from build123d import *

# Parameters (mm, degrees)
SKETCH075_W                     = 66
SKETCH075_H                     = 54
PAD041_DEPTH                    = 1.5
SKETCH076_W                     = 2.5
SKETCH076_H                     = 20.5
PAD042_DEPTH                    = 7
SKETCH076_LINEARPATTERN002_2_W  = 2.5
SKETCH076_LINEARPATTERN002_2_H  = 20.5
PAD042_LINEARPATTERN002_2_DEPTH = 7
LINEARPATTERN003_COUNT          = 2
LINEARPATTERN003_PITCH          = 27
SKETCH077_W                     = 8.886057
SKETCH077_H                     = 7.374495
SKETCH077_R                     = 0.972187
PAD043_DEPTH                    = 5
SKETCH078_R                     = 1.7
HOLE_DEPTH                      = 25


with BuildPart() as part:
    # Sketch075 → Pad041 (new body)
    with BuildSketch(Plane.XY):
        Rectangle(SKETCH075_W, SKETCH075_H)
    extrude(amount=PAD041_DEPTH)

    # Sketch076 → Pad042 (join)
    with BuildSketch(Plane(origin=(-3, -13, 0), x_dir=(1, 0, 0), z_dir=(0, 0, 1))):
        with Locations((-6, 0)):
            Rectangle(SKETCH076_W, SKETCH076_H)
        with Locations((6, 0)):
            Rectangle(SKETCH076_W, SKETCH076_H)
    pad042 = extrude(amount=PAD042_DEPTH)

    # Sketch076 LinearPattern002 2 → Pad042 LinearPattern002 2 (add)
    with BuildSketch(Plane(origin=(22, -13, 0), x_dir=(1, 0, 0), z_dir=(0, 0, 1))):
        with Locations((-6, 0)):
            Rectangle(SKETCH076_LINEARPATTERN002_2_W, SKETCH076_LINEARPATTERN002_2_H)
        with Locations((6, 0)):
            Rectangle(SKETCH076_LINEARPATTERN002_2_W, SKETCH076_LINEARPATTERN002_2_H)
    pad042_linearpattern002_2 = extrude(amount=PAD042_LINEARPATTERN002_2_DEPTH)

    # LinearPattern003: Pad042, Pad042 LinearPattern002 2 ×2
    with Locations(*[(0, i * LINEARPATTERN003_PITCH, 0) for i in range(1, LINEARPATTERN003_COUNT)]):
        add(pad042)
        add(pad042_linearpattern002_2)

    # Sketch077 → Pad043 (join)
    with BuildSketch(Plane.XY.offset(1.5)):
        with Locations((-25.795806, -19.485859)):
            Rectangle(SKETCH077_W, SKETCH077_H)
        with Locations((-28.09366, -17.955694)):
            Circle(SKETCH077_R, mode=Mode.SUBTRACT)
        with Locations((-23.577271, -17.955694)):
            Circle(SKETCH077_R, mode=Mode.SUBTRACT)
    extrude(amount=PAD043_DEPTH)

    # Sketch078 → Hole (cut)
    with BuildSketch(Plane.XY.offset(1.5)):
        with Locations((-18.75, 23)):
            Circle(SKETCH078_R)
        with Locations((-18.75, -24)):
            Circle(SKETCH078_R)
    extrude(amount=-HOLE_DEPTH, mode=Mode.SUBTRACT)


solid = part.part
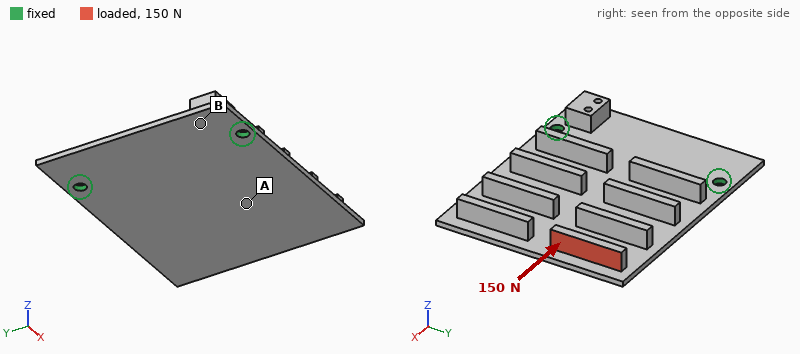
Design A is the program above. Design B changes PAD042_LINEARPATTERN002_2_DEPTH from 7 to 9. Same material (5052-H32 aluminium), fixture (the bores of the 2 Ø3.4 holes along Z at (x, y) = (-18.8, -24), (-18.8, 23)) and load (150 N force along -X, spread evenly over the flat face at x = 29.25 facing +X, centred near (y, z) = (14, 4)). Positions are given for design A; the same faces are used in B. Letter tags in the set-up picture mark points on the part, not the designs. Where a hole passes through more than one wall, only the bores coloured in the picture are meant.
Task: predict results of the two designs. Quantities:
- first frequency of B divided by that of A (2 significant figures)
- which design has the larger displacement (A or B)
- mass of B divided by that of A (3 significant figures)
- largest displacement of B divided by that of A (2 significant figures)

0.94
B
1.05
1.3
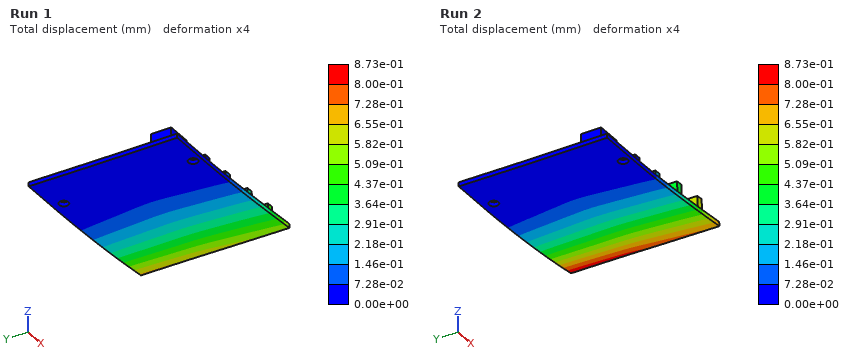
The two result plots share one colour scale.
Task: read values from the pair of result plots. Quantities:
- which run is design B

Run 2
